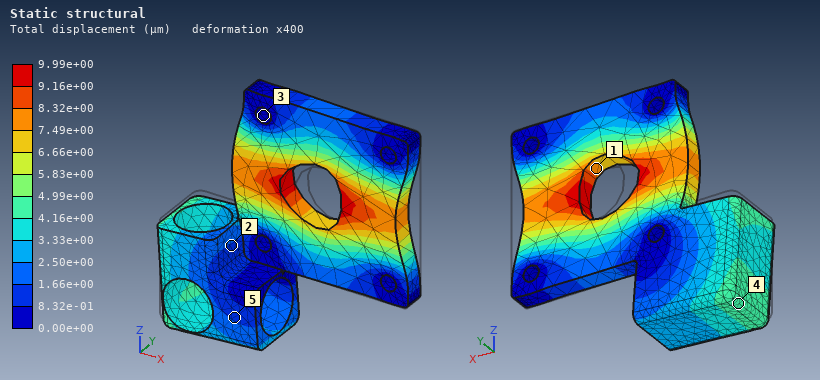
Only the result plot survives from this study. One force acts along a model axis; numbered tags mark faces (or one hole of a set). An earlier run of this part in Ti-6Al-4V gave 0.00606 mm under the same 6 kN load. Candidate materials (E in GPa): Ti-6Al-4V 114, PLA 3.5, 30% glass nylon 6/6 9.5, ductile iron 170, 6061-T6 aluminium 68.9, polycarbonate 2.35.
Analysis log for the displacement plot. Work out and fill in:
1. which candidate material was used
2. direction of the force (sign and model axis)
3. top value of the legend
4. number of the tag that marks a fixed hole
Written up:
6061-T6 aluminium
-X
9.99e+00 µm
3
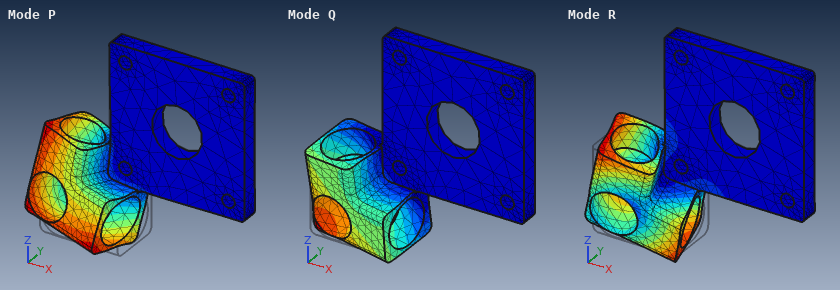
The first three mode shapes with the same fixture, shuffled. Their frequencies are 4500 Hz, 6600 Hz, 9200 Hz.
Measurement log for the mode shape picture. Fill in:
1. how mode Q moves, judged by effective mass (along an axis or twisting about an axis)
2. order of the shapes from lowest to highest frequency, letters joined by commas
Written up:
along Y
Q, P, R
